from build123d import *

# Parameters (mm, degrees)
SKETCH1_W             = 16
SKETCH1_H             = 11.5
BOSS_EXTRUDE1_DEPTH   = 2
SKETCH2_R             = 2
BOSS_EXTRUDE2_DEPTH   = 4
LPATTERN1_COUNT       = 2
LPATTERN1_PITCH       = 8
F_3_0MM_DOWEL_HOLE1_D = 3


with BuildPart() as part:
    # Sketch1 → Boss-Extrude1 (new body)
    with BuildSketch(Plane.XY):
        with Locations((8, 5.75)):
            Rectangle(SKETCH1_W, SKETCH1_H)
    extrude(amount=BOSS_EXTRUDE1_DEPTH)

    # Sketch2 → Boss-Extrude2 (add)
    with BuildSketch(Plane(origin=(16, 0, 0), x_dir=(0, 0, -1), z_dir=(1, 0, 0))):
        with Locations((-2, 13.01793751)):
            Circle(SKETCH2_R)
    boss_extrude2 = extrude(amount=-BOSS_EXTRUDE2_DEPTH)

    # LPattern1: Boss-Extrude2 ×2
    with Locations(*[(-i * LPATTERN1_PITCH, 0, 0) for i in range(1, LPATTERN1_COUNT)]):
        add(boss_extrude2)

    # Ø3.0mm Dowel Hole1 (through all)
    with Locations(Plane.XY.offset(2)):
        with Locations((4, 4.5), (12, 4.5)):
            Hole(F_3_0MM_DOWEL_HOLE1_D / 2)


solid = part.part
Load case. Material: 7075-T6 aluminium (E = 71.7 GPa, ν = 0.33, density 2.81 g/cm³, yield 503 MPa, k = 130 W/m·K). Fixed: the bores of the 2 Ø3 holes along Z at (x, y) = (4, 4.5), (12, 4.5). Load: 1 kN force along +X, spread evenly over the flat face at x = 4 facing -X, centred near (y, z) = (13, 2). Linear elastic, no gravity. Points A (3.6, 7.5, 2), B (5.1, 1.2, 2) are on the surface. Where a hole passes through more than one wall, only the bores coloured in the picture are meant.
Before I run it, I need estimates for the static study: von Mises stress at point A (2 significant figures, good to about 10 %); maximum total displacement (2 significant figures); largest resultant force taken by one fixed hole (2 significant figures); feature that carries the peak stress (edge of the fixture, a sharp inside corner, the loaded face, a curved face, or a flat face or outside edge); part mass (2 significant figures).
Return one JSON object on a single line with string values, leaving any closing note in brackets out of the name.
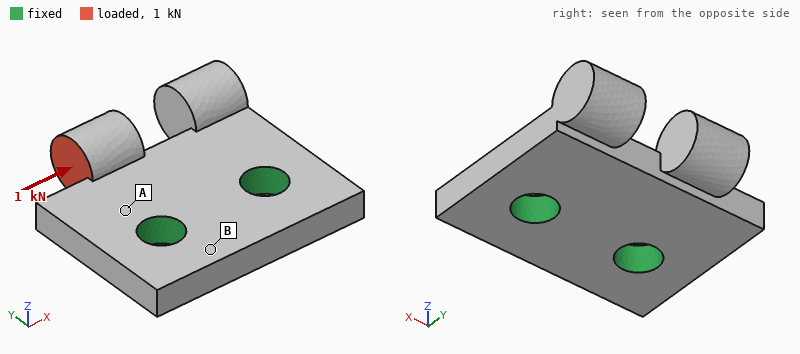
{"von Mises stress at point A": "120 MPa", "maximum total displacement": "60 µm", "largest resultant force taken by one fixed hole": "980 N", "feature that carries the peak stress": "a flat face or outside edge", "part mass": "1.2 g"}
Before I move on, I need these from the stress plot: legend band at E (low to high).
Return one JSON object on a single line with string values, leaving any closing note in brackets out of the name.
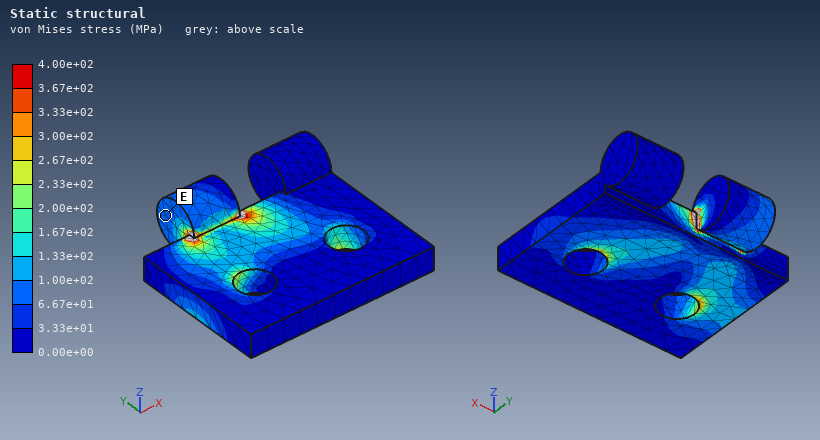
{"legend band at E": "6.67e+01 to 1.00e+02 MPa"}
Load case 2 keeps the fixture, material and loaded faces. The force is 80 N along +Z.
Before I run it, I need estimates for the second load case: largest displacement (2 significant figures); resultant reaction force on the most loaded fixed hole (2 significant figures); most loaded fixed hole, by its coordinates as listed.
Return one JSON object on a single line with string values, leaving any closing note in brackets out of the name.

{"largest displacement": "43 µm", "resultant reaction force on the most loaded fixed hole": "76 N", "most loaded fixed hole, by its coordinates as listed": "(4, 4.5)"}
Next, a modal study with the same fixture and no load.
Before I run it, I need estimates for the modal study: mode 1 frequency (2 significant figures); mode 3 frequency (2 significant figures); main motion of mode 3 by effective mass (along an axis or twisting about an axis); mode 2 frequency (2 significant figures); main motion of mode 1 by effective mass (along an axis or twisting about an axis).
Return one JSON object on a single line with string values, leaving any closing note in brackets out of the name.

{"mode 1 frequency": "17 kHz", "mode 3 frequency": "46 kHz", "main motion of mode 3 by effective mass": "along X", "mode 2 frequency": "22 kHz", "main motion of mode 1 by effective mass": "along Z"}
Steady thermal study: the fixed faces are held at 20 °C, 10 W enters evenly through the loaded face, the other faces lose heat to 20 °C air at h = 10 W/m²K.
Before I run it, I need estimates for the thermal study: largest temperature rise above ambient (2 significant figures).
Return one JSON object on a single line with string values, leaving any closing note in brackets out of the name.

{"largest temperature rise above ambient": "49 K"}
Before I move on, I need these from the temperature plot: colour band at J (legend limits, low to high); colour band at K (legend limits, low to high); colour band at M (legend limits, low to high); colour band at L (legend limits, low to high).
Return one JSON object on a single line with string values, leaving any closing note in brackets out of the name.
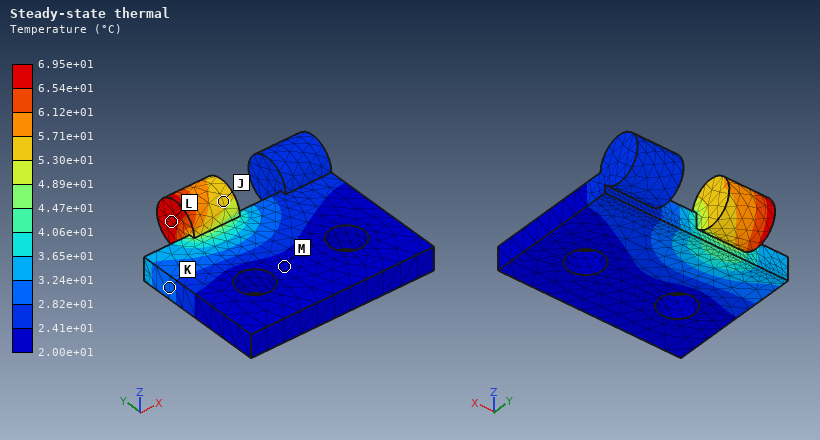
{"colour band at J": "5.30e+01 to 5.71e+01 °C", "colour band at K": "2.82e+01 to 3.24e+01 °C", "colour band at M": "2.00e+01 to 2.41e+01 °C", "colour band at L": "6.54e+01 to 6.95e+01 °C"}
